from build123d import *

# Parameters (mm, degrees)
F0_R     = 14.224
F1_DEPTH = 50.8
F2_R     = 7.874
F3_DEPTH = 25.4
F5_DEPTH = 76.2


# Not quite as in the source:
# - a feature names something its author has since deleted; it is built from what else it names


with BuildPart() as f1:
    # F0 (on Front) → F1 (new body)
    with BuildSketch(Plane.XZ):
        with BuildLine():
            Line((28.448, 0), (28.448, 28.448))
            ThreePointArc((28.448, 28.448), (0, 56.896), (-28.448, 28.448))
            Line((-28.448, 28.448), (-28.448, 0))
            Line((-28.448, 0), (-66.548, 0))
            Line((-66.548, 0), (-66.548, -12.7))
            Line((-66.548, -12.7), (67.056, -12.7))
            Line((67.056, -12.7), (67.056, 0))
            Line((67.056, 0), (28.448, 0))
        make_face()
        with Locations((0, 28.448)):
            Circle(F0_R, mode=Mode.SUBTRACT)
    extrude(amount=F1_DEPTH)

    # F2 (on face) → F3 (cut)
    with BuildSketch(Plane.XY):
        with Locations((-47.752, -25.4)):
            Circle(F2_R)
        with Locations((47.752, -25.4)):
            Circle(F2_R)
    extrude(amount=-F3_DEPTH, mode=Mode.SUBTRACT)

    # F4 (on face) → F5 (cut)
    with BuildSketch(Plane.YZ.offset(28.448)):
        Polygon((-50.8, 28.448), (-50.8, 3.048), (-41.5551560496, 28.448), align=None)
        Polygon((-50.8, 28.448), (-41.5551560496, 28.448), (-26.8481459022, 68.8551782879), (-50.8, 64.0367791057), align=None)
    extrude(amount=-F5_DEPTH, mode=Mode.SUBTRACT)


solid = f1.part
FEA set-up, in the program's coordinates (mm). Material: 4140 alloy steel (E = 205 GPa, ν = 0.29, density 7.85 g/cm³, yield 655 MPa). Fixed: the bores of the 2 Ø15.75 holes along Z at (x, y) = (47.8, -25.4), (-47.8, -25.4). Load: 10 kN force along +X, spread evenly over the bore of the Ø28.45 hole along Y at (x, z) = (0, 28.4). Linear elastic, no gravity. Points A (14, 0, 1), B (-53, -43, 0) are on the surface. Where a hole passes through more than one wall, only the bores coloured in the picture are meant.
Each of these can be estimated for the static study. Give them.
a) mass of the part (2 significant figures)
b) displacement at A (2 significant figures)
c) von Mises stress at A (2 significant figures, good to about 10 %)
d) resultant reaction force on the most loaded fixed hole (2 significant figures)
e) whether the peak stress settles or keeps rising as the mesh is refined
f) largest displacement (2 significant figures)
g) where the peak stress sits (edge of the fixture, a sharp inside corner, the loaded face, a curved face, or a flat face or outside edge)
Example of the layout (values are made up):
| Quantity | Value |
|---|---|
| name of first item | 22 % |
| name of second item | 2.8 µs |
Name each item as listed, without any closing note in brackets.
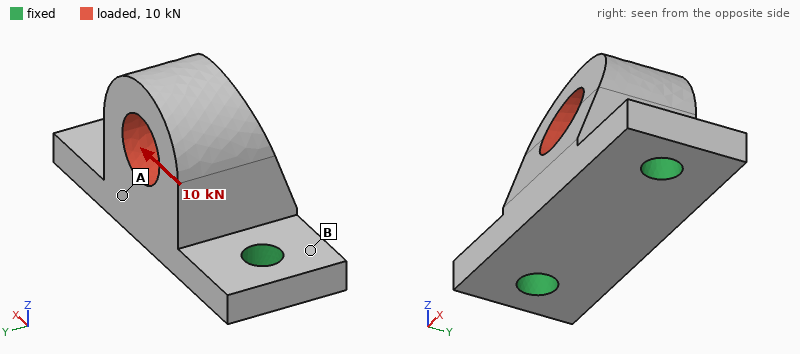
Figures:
| Quantity | Value |
|---|---|
| mass of the part | 1.4 kg |
| displacement at A | 2.7 µm |
| von Mises stress at A | 9.6 MPa |
| resultant reaction force on the most loaded fixed hole | 6.9 kN |
| whether the peak stress settles or keeps rising as the mesh is refined | keeps rising |
| largest displacement | 15 µm |
| where the peak stress sits | edge of the fixture |
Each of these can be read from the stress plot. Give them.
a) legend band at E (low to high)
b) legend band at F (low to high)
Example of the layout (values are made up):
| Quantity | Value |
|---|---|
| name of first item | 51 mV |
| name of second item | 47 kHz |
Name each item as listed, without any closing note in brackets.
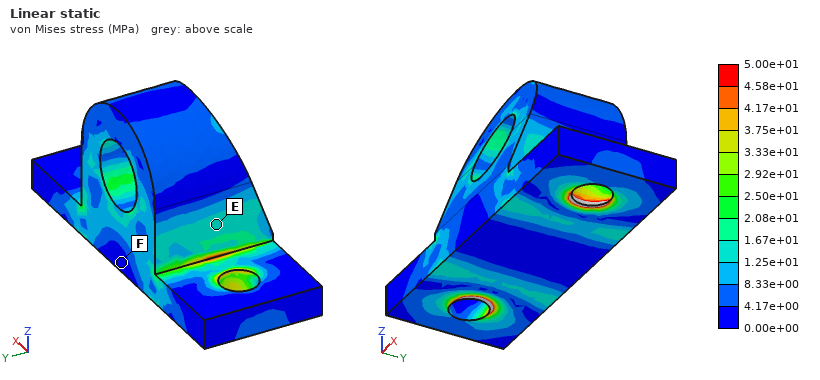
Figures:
| Quantity | Value |
|---|---|
| legend band at E | 1.25e+01 to 1.67e+01 MPa |
| legend band at F | 0.00e+00 to 4.17e+00 MPa |
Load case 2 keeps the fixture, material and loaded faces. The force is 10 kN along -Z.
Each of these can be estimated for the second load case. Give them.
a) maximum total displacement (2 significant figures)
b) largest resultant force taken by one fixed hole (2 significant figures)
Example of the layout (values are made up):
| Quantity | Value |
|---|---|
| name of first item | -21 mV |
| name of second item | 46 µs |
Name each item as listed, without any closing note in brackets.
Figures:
| Quantity | Value |
|---|---|
| maximum total displacement | 14 µm |
| largest resultant force taken by one fixed hole | 5.4 kN |
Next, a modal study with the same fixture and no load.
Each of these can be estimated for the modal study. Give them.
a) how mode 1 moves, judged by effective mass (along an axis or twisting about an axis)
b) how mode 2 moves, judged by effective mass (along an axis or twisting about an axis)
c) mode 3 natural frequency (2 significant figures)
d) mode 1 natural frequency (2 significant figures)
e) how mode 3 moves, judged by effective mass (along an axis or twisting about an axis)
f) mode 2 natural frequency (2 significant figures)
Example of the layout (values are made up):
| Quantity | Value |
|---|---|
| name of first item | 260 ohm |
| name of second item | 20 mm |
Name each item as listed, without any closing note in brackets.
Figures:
| Quantity | Value |
|---|---|
| how mode 1 moves, judged by effective mass | along Y |
| how mode 2 moves, judged by effective mass | along X |
| mode 3 natural frequency | 6200 Hz |
| mode 1 natural frequency | 2700 Hz |
| how mode 3 moves, judged by effective mass | along Z |
| mode 2 natural frequency | 5800 Hz |
